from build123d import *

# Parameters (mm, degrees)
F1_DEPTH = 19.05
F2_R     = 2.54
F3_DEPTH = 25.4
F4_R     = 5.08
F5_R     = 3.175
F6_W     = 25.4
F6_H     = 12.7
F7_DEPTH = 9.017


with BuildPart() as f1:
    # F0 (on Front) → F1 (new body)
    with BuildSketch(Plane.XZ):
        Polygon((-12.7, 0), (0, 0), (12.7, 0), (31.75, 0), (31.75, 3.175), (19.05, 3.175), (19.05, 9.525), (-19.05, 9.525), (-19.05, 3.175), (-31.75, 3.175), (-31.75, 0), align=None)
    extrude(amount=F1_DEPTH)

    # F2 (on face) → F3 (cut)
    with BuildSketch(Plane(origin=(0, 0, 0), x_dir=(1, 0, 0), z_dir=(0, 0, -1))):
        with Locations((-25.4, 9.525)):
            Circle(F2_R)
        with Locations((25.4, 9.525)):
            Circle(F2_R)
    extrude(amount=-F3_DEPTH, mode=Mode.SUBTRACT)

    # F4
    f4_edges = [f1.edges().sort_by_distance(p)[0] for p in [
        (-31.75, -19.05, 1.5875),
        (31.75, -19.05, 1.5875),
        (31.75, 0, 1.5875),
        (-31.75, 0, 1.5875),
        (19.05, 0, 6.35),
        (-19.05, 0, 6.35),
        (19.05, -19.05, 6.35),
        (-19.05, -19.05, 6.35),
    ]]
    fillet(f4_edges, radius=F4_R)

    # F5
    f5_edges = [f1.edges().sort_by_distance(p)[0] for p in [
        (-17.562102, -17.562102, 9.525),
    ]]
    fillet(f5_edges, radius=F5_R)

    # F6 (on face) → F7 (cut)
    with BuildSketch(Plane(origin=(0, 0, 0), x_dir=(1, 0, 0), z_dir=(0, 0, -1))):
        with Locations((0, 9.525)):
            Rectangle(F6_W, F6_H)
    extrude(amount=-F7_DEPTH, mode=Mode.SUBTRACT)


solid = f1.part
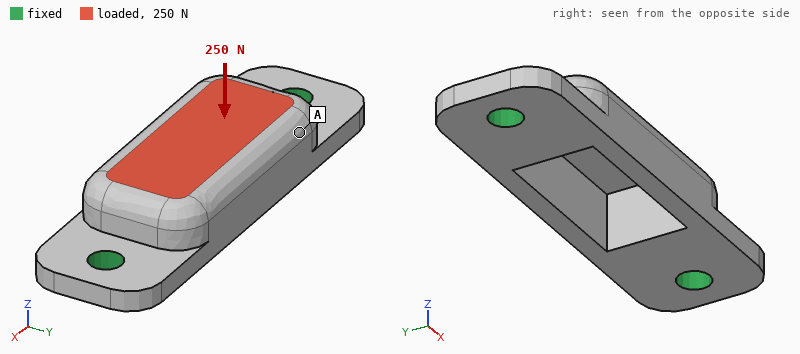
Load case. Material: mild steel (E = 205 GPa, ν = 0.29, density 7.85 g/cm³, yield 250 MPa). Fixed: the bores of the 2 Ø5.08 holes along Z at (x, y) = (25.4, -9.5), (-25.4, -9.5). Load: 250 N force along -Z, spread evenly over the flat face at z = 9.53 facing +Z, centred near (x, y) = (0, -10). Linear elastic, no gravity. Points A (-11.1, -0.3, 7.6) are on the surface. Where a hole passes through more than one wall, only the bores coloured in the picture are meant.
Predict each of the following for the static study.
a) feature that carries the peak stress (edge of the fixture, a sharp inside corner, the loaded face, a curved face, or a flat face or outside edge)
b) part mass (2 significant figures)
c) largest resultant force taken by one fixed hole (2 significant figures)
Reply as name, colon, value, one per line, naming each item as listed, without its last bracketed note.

feature that carries the peak stress: the loaded face
part mass: 39 g
largest resultant force taken by one fixed hole: 190 N
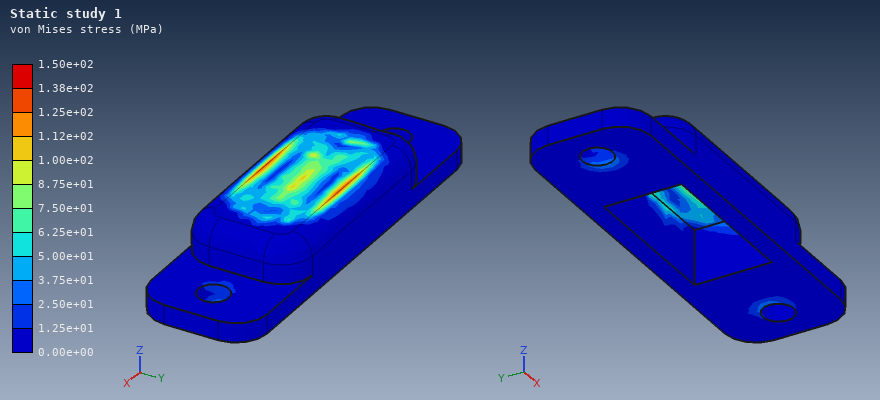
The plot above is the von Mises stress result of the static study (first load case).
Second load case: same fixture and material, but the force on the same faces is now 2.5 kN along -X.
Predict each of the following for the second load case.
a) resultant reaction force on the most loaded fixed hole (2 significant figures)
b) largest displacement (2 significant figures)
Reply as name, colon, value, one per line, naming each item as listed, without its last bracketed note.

resultant reaction force on the most loaded fixed hole: 1.3 kN
largest displacement: 6.3 µm
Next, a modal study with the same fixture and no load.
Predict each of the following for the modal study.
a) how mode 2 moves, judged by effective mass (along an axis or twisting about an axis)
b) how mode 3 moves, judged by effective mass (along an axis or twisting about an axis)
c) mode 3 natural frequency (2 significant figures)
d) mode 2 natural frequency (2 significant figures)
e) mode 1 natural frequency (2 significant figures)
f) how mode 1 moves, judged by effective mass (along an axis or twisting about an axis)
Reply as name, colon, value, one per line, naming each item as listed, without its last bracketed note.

how mode 2 moves, judged by effective mass: along Z
how mode 3 moves, judged by effective mass: along Y
mode 3 natural frequency: 18 kHz
mode 2 natural frequency: 12 kHz
mode 1 natural frequency: 9200 Hz
how mode 1 moves, judged by effective mass: along Y
